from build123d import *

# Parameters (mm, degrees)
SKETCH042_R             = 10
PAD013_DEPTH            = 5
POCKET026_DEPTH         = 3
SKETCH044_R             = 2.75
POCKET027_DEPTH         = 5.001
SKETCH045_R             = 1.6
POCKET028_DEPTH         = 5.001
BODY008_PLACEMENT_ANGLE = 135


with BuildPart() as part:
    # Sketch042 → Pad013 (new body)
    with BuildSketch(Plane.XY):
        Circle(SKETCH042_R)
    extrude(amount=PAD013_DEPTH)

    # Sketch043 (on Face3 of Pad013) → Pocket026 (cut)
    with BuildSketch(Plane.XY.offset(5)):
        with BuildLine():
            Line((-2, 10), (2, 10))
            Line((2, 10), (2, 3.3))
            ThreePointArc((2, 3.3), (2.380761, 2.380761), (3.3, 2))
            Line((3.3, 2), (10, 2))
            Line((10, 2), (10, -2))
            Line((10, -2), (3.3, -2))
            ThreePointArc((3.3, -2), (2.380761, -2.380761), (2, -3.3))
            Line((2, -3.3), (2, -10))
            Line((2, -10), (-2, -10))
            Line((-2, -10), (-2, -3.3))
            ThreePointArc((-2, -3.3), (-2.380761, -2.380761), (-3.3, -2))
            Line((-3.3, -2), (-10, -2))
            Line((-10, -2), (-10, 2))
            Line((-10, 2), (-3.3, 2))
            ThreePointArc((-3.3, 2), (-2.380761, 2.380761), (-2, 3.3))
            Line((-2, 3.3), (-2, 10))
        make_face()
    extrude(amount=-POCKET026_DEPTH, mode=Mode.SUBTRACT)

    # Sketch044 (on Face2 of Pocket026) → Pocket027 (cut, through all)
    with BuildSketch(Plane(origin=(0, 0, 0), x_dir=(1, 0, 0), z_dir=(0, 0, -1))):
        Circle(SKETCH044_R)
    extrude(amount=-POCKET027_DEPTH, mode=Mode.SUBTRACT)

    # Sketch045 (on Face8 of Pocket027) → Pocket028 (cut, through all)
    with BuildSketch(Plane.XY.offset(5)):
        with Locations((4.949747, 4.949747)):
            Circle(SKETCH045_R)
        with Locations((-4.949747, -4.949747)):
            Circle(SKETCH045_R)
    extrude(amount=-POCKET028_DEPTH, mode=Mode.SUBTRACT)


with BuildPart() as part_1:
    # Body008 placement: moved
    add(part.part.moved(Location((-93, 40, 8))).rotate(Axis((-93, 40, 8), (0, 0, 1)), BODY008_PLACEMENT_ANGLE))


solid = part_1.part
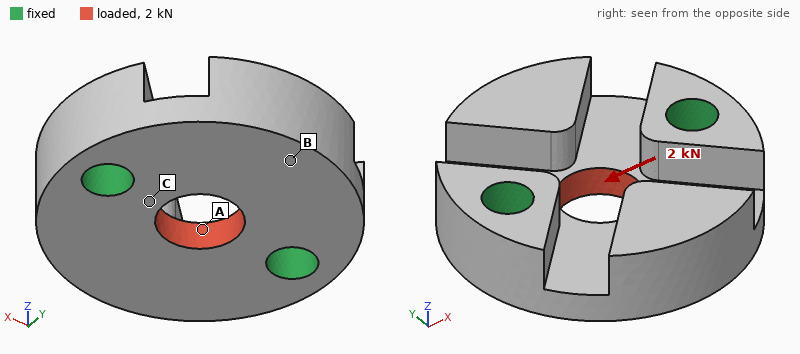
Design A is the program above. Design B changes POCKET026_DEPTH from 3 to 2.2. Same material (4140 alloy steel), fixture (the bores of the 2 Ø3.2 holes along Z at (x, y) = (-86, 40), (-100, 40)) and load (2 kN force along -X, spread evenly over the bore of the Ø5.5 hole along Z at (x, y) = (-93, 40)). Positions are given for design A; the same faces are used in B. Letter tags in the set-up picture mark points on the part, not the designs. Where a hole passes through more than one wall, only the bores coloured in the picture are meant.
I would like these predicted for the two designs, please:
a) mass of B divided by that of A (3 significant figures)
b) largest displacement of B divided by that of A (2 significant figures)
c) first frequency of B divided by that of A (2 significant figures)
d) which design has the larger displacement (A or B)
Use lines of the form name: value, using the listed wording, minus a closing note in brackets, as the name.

mass of B divided by that of A: 1.10
largest displacement of B divided by that of A: 0.73
first frequency of B divided by that of A: 1.4
which design has the larger displacement: A
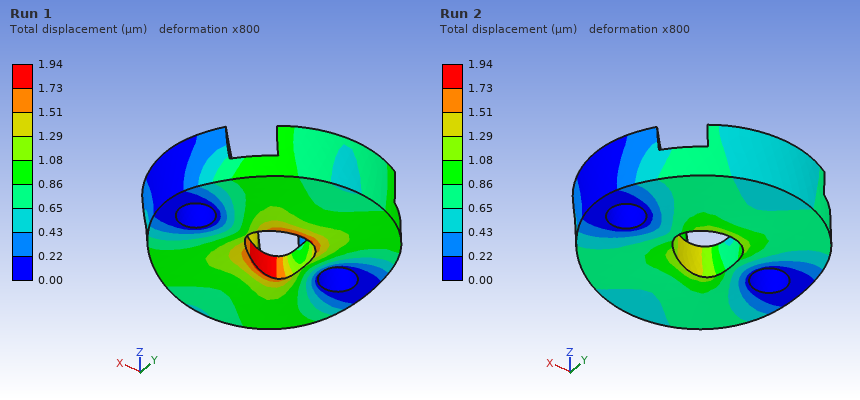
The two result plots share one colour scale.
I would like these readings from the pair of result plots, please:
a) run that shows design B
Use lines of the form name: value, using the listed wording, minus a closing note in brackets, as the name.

run that shows design B: Run 2
